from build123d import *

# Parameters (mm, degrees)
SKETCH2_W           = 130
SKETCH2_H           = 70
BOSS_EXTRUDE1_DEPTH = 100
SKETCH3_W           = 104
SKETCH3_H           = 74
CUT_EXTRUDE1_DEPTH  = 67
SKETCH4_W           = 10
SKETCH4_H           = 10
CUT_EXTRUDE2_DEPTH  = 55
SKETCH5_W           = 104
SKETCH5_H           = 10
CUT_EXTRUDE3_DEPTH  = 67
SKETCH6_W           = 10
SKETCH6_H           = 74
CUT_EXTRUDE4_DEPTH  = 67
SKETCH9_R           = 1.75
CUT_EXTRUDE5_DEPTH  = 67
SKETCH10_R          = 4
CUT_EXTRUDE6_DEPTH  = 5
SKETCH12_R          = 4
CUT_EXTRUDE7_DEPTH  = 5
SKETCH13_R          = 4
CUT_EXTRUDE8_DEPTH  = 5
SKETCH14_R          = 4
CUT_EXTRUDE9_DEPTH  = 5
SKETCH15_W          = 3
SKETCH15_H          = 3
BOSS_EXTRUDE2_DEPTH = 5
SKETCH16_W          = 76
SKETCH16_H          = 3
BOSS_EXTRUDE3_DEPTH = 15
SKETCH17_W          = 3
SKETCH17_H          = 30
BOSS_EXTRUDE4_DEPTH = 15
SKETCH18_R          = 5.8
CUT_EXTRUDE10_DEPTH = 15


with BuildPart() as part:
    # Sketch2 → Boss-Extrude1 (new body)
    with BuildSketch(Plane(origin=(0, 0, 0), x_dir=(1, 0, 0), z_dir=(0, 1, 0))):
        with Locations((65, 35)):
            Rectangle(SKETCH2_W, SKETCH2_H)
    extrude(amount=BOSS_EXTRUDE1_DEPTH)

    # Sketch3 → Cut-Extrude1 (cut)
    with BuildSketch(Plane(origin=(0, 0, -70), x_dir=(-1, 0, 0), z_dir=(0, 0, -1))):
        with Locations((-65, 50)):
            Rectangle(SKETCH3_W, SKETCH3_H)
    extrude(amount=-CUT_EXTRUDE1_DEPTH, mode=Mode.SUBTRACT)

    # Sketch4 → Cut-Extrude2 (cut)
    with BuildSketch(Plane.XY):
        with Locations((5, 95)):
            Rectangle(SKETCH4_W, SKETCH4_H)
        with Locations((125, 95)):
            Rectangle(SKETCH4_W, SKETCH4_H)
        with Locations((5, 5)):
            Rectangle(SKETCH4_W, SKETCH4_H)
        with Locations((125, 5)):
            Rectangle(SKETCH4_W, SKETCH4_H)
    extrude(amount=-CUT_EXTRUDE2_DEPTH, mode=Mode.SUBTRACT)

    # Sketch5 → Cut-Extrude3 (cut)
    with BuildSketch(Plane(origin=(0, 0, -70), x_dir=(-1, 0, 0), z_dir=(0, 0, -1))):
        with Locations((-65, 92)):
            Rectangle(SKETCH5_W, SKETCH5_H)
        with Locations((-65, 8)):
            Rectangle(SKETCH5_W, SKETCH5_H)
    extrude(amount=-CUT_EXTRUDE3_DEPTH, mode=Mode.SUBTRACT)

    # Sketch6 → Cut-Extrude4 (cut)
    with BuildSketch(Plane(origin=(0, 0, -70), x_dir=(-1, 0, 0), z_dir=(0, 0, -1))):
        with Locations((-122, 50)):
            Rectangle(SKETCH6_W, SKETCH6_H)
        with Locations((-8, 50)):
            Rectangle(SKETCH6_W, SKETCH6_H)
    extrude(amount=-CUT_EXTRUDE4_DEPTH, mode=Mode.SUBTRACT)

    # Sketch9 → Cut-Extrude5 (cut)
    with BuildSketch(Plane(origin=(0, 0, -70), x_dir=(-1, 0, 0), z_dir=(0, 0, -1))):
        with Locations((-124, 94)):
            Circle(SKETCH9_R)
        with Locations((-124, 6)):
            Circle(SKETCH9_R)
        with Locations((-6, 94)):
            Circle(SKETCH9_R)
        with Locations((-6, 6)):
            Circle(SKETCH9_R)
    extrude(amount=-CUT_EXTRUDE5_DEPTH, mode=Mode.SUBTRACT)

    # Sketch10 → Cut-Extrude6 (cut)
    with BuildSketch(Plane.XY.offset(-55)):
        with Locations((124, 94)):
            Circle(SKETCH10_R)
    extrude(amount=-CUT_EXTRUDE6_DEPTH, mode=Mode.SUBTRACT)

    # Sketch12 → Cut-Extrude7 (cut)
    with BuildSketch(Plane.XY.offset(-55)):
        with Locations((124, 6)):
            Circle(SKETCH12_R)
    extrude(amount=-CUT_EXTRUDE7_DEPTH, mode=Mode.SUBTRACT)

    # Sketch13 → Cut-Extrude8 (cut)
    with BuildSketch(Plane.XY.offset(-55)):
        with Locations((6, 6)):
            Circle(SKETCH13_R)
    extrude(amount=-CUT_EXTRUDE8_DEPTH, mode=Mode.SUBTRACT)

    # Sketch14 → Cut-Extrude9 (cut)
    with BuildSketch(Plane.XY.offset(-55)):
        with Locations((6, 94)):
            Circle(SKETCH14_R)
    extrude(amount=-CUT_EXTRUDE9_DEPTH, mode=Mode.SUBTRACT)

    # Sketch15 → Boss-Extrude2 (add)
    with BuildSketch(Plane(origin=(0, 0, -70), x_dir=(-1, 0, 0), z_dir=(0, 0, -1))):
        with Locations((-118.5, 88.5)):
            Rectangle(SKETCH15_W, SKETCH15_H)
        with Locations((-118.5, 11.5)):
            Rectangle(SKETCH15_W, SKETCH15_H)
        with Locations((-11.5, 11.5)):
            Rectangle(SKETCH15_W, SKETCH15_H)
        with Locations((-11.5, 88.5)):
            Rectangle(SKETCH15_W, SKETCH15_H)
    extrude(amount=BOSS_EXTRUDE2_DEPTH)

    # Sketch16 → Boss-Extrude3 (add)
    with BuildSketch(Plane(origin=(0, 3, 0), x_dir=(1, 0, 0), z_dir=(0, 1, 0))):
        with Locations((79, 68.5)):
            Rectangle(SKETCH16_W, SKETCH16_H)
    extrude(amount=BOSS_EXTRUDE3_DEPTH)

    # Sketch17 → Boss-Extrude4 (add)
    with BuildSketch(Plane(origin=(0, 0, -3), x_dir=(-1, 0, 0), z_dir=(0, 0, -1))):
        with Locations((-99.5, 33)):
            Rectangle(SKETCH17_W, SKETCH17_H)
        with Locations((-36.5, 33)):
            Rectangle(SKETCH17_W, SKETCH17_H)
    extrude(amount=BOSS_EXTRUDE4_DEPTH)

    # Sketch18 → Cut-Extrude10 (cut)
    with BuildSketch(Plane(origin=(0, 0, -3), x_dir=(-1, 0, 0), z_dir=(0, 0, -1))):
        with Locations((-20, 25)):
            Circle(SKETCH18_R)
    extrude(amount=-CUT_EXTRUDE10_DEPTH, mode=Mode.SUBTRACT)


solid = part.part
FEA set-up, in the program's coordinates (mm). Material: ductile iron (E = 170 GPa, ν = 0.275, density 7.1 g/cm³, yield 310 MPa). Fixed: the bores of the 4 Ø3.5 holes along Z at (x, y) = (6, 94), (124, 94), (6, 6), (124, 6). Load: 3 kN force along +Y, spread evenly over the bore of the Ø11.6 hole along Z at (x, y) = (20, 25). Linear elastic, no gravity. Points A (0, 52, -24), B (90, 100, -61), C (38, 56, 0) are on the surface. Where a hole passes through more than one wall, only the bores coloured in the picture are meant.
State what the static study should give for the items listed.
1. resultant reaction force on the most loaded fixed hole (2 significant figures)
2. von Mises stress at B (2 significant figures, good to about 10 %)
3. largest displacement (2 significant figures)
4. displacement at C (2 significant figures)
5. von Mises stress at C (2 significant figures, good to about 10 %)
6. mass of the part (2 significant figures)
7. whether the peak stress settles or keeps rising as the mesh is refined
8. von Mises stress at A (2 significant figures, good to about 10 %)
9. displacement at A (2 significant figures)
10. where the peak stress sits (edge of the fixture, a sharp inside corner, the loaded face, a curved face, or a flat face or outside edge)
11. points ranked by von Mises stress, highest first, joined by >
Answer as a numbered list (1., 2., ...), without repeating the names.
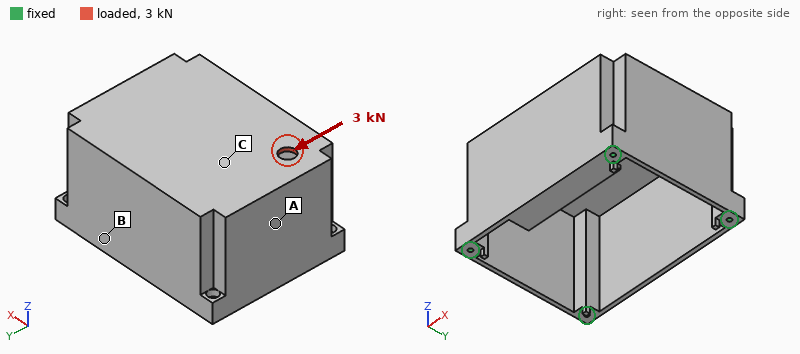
1. 1.7 kN
2. 2.5 MPa
3. 17 µm
4. 13 µm
5. 7.7 MPa
6. 980 g
7. keeps rising
8. 17 MPa
9. 7.9 µm
10. edge of the fixture
11. A > C > B
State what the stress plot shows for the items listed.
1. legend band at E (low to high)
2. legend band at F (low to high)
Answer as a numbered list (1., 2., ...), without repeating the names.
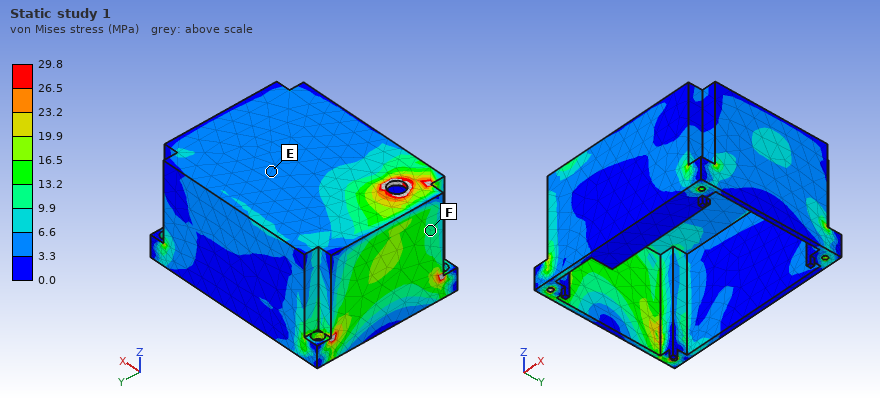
1. 3.3 to 6.6 MPa
2. 9.9 to 13.2 MPa
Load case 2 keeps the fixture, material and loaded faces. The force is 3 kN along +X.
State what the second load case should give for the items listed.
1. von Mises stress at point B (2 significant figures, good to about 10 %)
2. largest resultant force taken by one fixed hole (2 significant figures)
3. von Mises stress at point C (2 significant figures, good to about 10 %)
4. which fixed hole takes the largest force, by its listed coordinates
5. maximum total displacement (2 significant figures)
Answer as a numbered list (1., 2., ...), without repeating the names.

1. 3.4 MPa
2. 1.4 kN
3. 8.1 MPa
4. (124, 6)
5. 14 µm
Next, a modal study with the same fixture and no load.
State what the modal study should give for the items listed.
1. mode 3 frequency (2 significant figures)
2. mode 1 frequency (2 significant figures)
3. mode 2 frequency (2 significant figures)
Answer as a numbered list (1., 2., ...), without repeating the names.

1. 2100 Hz
2. 1500 Hz
3. 1700 Hz
